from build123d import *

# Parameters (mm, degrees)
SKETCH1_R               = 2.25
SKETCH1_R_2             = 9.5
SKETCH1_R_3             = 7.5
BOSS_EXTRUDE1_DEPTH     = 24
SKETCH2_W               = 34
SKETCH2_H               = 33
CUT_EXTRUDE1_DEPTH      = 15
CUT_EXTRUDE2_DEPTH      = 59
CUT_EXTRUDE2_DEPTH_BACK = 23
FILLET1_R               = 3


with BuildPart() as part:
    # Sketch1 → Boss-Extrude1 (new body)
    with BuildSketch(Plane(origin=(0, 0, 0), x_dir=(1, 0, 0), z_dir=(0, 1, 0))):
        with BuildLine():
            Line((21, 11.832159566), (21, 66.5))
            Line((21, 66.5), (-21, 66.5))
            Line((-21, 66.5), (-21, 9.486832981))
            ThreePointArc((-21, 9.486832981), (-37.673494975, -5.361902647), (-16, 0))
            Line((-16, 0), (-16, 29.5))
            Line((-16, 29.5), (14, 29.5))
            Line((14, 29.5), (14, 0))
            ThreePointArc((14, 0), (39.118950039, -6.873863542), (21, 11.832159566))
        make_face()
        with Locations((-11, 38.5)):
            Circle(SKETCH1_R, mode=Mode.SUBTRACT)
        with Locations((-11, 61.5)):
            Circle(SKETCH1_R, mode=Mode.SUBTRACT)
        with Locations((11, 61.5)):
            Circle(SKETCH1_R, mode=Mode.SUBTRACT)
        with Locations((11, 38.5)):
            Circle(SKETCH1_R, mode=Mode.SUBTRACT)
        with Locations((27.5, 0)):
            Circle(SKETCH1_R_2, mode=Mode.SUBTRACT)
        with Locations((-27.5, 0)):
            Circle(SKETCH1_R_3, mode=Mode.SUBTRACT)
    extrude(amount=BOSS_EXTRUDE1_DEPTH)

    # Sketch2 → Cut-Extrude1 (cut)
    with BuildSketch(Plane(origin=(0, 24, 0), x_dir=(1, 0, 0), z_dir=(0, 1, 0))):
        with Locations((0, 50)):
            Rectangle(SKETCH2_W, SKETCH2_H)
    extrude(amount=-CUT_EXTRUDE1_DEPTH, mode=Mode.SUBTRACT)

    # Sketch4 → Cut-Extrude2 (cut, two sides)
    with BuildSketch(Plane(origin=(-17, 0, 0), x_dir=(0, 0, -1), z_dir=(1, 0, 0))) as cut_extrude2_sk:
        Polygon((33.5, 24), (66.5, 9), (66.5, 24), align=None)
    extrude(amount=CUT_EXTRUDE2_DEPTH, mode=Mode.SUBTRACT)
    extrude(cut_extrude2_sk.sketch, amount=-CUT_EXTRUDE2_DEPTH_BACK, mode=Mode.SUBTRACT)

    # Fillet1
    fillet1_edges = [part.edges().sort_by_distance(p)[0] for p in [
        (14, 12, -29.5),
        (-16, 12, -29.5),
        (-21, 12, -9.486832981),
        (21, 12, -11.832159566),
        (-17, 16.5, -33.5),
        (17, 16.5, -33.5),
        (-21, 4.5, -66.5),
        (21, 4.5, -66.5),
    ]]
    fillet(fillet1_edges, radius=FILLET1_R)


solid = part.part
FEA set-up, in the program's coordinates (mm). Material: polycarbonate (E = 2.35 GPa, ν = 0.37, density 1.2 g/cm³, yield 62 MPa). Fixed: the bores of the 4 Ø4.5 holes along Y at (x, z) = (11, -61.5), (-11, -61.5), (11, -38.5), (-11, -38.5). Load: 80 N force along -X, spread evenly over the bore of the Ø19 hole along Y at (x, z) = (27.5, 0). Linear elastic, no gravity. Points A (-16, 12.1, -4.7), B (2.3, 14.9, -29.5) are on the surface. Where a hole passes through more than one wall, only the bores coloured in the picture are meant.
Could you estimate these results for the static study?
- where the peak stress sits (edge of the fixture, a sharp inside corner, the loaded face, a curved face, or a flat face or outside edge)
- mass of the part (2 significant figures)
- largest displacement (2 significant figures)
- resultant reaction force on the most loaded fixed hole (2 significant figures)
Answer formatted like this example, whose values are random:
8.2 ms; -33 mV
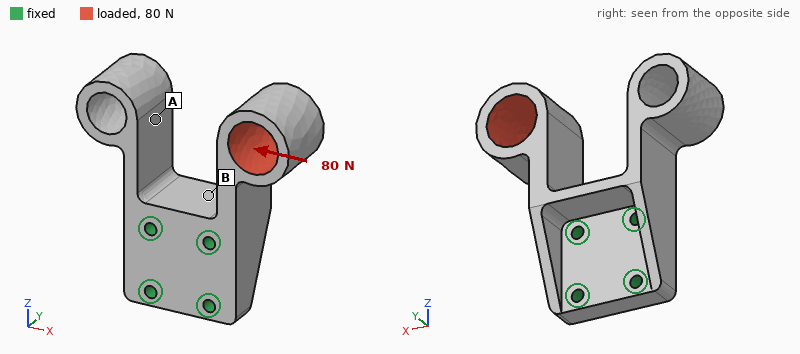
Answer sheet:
a curved face; 45 g; 1.2 mm; 92 N
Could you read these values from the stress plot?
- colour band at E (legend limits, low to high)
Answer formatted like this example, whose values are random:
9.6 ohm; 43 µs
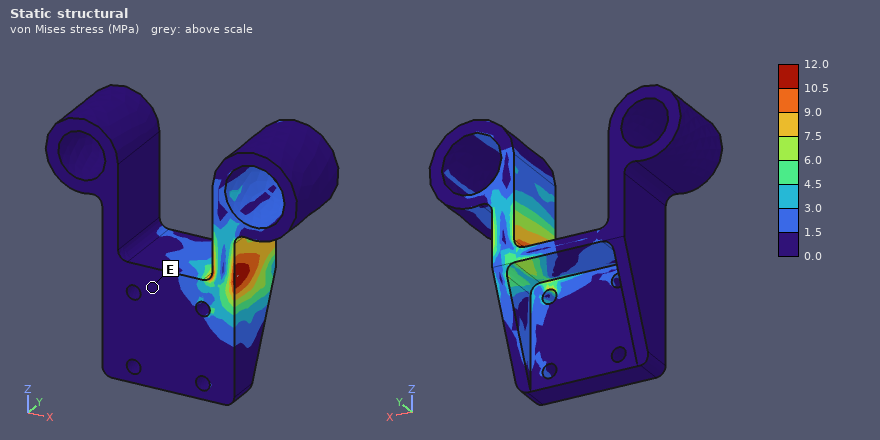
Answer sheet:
0.0 to 1.5 MPa
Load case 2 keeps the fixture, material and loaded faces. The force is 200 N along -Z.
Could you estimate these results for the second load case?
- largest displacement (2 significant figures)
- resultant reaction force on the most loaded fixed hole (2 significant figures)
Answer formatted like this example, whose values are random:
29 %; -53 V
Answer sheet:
1.3 mm; 140 N
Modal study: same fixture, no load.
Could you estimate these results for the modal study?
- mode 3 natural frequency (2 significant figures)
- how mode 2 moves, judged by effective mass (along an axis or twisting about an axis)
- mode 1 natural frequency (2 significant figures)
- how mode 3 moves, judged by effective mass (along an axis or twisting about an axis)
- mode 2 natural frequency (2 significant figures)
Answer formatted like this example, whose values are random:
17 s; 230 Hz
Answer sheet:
760 Hz; along X; 380 Hz; twisting about Z; 480 Hz
